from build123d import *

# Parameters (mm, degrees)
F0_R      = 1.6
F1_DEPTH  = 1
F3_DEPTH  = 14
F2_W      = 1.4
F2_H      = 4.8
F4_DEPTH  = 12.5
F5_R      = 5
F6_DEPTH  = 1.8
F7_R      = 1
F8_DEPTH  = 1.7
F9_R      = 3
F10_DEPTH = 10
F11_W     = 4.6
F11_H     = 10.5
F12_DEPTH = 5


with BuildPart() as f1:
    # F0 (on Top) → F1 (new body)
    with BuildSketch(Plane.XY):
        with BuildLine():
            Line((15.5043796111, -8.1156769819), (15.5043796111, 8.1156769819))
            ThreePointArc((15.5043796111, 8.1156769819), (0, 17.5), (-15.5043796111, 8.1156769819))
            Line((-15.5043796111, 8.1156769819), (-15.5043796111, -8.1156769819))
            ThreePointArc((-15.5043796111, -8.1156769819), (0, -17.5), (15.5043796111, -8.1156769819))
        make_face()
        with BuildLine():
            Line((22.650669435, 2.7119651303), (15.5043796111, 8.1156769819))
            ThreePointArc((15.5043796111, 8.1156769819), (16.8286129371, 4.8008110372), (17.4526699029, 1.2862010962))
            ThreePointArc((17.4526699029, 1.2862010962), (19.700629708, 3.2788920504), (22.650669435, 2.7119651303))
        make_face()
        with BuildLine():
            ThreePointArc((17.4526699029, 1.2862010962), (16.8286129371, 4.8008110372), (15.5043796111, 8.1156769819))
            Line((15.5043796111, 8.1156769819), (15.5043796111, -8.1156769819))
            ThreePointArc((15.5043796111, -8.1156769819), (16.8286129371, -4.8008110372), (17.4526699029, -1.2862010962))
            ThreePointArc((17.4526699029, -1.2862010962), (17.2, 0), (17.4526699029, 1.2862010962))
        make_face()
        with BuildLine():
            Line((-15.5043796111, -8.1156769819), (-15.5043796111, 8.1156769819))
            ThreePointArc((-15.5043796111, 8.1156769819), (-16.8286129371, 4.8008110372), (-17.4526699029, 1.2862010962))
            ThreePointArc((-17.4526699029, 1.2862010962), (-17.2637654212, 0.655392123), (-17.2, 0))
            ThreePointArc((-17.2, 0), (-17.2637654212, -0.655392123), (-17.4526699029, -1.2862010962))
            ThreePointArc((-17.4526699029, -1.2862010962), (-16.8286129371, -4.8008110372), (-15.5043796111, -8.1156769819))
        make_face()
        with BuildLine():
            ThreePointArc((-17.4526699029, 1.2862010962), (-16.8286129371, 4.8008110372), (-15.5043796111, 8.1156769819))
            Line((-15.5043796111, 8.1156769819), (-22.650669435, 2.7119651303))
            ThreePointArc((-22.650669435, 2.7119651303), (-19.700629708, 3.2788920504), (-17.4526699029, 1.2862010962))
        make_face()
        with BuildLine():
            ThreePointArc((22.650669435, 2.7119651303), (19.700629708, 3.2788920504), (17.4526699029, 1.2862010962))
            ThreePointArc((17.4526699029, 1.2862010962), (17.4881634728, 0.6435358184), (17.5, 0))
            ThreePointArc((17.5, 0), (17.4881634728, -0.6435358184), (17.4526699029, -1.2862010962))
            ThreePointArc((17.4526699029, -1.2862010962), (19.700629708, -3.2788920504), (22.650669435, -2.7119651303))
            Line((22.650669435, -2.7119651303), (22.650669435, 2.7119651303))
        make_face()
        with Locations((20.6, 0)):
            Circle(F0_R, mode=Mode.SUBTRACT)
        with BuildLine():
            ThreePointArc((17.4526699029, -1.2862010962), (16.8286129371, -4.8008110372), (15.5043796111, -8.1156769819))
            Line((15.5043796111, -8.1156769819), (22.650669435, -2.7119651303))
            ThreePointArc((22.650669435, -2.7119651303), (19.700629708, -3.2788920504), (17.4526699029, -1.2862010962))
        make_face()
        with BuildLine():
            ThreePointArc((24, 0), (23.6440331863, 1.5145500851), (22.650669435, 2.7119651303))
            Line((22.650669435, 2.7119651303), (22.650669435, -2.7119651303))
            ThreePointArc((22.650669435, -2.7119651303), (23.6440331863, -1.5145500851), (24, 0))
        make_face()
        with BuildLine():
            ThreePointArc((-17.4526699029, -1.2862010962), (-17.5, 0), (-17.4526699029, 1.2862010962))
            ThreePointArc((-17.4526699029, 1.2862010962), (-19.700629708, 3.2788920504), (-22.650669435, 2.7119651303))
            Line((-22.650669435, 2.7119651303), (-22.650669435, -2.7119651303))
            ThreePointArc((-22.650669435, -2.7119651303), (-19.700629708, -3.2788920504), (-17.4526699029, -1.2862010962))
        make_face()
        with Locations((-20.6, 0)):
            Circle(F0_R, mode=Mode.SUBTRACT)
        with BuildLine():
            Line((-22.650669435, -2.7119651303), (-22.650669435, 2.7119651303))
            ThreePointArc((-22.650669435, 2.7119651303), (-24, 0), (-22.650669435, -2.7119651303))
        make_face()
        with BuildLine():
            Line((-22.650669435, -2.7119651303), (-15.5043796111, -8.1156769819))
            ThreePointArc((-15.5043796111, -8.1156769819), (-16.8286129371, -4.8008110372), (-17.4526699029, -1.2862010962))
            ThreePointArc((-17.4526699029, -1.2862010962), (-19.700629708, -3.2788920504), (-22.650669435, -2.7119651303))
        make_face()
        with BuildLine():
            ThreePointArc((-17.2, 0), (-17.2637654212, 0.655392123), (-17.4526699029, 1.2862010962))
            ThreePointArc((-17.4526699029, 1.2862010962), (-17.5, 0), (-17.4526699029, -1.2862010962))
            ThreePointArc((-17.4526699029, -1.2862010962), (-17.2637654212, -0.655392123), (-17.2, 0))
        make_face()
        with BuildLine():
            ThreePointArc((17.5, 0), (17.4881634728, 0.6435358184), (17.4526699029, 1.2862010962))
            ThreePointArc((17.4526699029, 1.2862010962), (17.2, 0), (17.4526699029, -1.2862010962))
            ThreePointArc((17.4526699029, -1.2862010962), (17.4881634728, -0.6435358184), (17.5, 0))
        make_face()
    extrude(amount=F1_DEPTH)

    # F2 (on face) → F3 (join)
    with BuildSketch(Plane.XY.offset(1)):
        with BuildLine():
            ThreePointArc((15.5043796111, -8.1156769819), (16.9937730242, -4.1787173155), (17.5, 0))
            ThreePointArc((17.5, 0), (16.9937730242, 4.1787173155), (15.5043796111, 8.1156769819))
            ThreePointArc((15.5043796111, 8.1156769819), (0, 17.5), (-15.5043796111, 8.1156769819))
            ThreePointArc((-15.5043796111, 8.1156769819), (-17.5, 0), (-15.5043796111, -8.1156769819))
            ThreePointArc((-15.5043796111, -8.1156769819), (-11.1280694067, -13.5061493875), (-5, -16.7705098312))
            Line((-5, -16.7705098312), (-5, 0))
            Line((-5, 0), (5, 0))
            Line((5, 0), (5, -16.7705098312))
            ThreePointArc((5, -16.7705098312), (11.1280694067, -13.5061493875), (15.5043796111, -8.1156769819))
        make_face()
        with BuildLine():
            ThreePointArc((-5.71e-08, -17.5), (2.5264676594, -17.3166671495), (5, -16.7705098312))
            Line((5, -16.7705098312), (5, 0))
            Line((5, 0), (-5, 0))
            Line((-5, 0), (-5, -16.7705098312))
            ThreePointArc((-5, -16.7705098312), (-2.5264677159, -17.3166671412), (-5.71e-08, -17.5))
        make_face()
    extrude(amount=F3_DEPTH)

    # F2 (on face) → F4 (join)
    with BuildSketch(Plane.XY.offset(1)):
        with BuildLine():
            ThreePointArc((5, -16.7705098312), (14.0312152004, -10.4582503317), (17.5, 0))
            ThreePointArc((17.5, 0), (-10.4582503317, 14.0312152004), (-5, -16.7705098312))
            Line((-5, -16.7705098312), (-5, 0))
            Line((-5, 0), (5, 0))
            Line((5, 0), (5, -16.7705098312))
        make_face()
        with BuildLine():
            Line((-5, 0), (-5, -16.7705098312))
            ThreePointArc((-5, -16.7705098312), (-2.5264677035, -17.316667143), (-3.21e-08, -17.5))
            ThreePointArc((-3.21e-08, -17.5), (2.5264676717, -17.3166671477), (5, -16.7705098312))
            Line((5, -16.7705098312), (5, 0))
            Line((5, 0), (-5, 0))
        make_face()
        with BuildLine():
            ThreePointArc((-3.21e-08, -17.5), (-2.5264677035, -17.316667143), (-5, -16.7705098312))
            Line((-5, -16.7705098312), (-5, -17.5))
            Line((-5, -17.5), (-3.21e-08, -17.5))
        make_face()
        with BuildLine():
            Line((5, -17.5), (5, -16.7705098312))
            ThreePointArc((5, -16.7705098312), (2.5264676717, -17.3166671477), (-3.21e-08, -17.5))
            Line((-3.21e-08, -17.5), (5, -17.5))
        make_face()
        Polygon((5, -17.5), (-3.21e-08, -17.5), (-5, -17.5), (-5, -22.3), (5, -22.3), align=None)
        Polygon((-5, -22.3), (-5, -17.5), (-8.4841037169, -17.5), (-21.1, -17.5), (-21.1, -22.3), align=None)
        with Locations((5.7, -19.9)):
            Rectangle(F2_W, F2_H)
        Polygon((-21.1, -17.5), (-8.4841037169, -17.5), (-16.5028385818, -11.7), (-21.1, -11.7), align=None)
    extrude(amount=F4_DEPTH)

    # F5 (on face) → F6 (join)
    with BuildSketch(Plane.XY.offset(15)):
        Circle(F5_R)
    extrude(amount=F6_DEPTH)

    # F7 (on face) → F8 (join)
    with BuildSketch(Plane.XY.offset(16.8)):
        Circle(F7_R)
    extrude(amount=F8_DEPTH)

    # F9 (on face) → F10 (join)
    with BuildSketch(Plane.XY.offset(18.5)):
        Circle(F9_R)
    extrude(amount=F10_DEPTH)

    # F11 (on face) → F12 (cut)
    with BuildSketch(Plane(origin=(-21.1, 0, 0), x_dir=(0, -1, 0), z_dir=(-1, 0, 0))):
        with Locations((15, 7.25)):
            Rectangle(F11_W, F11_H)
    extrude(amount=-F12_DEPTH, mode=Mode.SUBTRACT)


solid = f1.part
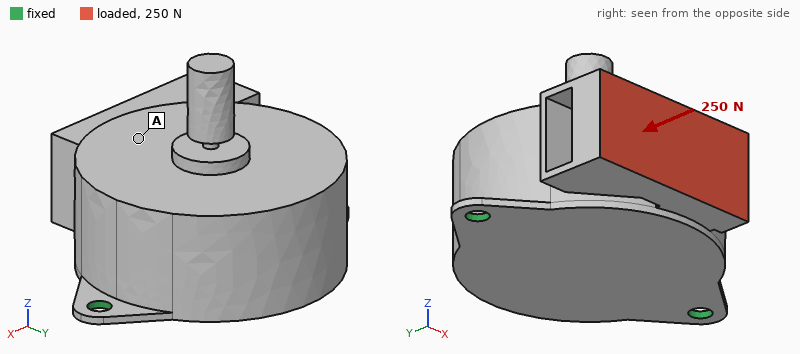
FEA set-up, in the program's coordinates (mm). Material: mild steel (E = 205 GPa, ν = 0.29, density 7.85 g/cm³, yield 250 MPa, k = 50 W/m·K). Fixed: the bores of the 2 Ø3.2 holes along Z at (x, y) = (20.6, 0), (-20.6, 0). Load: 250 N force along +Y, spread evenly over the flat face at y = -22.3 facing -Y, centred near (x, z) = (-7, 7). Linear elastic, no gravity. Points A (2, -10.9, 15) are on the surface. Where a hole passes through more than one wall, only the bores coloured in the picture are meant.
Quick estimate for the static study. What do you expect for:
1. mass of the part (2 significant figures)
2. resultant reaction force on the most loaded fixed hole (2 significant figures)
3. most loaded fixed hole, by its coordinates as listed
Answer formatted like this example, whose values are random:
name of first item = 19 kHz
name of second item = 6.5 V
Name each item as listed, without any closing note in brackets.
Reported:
mass of the part = 130 g
resultant reaction force on the most loaded fixed hole = 170 N
most loaded fixed hole, by its coordinates as listed = (-20.6, 0)
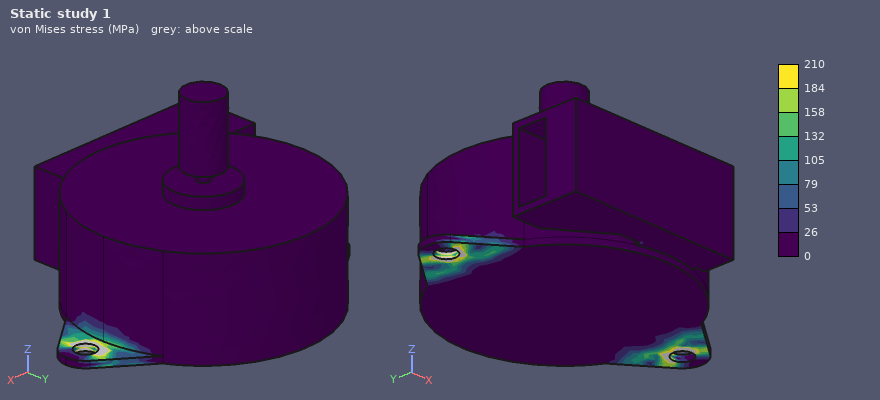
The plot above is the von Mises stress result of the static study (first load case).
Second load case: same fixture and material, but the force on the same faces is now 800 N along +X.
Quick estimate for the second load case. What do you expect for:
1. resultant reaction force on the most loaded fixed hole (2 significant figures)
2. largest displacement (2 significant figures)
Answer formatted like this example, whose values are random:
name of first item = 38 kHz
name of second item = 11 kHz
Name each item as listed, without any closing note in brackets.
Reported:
resultant reaction force on the most loaded fixed hole = 620 N
largest displacement = 15 µm
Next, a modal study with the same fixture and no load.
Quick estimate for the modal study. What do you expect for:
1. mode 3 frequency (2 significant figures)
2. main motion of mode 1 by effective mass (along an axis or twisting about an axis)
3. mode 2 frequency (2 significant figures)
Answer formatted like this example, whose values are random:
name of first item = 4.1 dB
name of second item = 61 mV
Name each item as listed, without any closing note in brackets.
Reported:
mode 3 frequency = 4000 Hz
main motion of mode 1 by effective mass = along Y
mode 2 frequency = 3900 Hz
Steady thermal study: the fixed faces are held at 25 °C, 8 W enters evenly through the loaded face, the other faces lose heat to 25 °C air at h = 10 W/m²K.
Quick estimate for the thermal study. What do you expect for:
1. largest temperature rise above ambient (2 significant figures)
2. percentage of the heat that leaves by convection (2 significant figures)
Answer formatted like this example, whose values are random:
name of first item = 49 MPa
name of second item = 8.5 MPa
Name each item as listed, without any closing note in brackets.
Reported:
largest temperature rise above ambient = 53 K
percentage of the heat that leaves by convection = 19 %
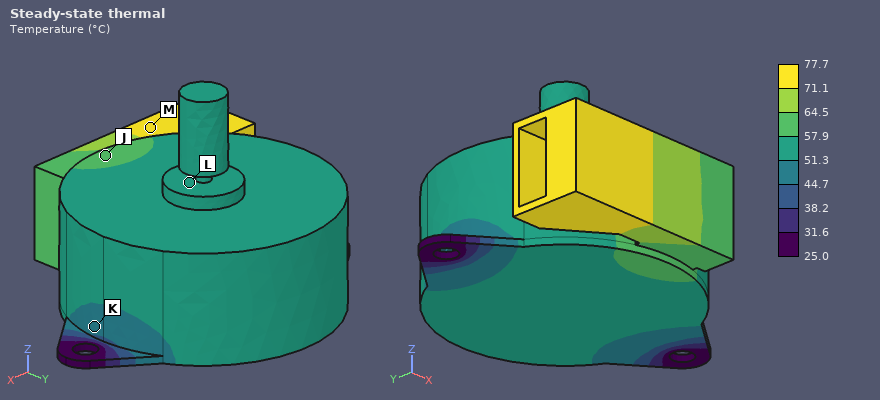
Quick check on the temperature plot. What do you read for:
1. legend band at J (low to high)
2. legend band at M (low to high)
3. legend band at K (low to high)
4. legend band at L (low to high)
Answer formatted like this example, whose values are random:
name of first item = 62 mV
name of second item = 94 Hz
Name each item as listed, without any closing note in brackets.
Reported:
legend band at J = 57.9 to 64.5 °C
legend band at M = 71.1 to 77.7 °C
legend band at K = 44.7 to 51.3 °C
legend band at L = 51.3 to 57.9 °C
